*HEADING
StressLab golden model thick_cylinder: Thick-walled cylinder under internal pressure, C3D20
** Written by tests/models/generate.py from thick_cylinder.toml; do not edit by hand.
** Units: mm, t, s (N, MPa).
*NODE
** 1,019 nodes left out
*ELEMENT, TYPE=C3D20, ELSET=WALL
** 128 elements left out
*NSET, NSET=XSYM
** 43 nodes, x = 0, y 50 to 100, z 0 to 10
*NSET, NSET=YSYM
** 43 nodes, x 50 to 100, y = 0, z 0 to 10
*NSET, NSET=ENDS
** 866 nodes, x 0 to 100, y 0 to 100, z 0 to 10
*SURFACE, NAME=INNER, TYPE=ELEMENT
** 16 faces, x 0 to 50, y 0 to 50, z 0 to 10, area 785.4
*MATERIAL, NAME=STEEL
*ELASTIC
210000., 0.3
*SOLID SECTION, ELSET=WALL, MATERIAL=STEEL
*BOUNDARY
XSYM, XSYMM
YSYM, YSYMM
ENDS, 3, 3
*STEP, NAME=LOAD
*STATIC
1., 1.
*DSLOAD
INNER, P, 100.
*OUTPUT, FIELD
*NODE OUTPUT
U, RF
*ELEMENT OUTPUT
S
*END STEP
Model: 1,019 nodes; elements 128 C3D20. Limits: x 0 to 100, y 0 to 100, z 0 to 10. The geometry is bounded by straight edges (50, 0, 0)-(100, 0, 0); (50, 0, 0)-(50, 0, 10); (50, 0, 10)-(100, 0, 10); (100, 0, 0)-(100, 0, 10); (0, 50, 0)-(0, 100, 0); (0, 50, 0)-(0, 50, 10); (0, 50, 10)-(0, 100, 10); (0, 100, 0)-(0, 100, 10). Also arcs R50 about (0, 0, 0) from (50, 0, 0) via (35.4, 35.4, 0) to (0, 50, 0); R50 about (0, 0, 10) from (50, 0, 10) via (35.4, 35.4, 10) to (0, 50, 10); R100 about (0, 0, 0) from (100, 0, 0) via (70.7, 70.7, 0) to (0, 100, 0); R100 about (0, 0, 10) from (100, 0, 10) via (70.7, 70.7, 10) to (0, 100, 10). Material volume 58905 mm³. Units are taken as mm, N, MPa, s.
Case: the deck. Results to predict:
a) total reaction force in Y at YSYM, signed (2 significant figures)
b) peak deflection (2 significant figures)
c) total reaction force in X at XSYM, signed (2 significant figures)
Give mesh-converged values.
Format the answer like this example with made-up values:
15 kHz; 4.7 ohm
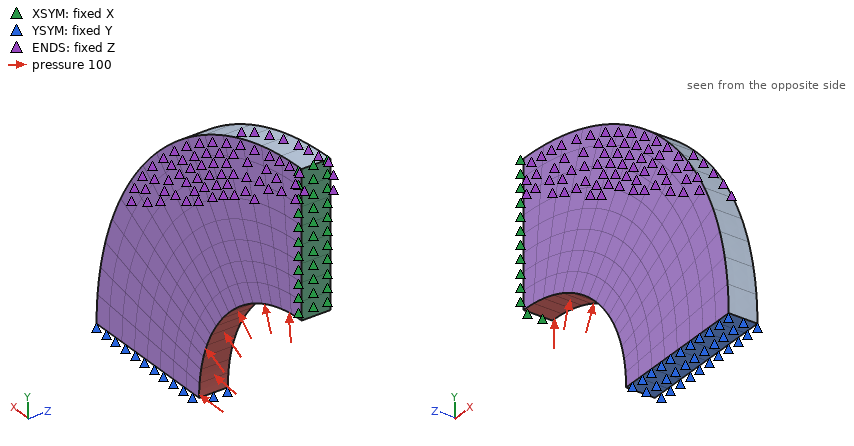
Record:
-50000 N; 0.045 mm; -50000 N
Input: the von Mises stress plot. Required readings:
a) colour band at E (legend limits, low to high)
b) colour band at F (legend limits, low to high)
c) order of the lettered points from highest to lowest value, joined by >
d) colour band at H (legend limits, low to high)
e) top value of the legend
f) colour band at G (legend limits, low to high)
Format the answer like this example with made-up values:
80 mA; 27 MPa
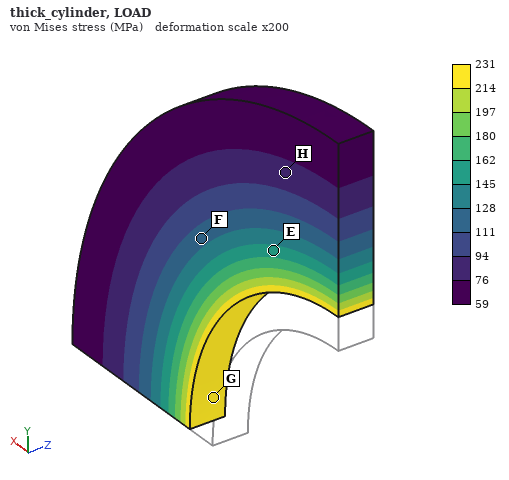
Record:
145 to 162 MPa; 111 to 128 MPa; G > E > F > H; 76 to 94 MPa; 231 MPa; 214 to 231 MPa
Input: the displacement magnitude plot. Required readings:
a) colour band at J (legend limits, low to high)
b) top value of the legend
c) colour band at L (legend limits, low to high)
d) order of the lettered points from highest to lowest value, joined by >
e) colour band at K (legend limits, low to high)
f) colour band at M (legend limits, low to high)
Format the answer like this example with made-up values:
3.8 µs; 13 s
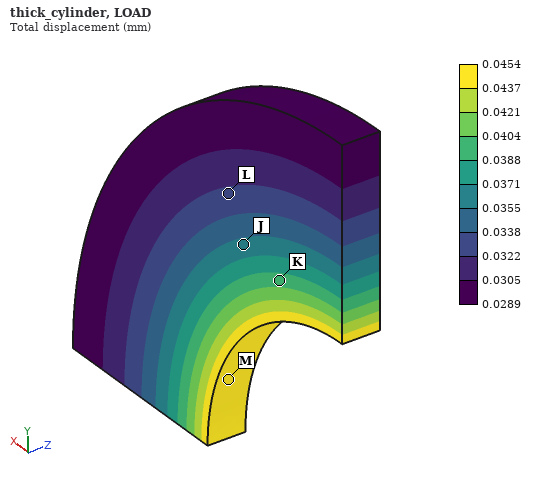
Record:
0.0355 to 0.0371 mm; 0.0454 mm; 0.0322 to 0.0338 mm; M > K > J > L; 0.0388 to 0.0404 mm; 0.0437 to 0.0454 mm
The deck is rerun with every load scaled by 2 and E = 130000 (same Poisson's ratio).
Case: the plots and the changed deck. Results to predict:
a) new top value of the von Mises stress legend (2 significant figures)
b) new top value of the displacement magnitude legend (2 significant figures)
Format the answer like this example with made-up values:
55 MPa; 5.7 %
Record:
460 MPa; 0.15 mm
